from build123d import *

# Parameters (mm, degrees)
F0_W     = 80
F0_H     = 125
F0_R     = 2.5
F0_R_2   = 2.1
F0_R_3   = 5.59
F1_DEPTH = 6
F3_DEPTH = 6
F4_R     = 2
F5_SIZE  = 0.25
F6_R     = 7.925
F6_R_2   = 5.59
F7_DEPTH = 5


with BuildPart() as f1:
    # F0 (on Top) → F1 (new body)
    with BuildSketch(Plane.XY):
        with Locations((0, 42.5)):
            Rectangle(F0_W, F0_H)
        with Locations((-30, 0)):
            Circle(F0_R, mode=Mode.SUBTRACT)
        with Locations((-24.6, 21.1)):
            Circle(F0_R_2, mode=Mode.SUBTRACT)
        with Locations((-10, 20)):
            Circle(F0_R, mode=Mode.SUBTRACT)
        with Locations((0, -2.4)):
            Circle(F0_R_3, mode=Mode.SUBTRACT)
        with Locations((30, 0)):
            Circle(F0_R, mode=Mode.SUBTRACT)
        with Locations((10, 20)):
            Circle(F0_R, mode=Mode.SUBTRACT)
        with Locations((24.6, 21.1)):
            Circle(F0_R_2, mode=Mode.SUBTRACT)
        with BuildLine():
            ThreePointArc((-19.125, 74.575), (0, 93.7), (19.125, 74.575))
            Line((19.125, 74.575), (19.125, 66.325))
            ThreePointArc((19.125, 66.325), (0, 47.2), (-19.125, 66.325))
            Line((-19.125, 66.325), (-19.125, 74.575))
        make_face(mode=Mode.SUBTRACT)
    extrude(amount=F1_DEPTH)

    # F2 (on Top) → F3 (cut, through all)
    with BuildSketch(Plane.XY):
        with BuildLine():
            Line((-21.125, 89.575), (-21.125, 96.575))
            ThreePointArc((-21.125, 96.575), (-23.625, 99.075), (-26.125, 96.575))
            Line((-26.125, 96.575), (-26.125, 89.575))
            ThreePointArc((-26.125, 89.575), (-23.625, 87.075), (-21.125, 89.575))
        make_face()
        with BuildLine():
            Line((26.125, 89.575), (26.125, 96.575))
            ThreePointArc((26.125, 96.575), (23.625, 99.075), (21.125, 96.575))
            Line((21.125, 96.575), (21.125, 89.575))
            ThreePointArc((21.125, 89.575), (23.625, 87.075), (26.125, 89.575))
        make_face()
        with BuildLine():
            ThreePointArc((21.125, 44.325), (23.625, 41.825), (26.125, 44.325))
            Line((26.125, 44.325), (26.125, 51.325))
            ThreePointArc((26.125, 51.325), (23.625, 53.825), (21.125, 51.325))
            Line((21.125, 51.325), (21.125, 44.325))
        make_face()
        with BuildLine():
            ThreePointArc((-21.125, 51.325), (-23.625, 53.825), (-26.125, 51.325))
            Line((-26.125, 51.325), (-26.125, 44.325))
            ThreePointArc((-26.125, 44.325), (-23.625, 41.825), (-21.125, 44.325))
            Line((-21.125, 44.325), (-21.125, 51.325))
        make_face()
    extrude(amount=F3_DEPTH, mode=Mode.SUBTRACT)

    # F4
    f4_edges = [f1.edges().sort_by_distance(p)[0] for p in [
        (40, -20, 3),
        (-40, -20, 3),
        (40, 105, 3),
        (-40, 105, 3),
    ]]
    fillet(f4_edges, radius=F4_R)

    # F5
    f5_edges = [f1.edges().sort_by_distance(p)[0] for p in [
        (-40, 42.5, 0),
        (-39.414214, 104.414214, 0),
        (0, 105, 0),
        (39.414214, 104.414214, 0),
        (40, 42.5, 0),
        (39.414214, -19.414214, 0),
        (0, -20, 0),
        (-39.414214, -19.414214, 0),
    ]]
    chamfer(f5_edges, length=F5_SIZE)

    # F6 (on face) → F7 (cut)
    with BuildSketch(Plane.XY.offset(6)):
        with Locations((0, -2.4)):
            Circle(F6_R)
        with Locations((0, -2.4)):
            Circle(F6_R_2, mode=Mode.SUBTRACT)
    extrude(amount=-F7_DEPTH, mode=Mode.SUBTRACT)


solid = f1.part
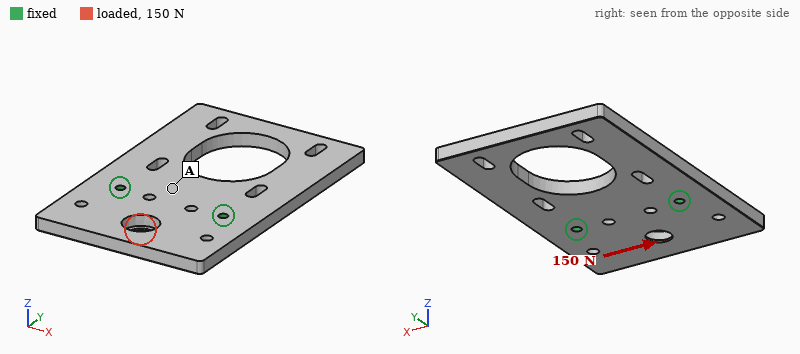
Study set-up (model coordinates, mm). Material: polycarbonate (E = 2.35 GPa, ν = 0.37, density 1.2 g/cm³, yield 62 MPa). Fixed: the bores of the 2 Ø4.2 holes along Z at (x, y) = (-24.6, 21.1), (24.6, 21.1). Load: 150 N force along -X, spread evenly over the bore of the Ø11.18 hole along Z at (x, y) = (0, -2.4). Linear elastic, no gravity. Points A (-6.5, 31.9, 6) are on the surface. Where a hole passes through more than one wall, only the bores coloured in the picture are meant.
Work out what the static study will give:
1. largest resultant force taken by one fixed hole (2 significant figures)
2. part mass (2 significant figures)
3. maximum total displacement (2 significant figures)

100 N
58 g
45 µm
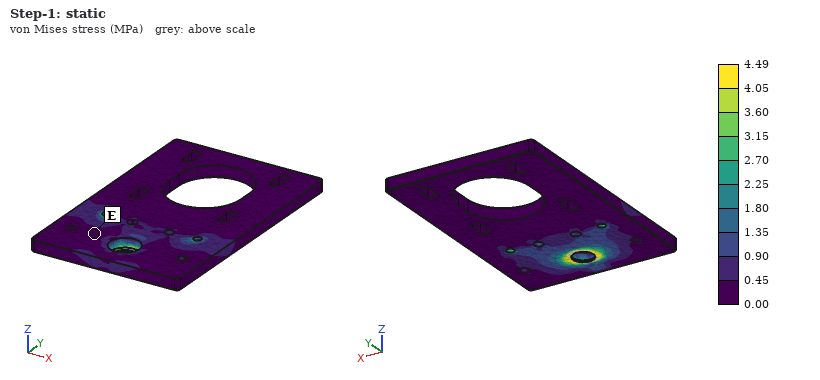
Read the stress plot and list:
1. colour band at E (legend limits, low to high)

0.00 to 0.45 MPa
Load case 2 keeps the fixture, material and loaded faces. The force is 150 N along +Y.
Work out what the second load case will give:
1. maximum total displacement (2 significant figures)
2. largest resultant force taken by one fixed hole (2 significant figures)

0.11 mm
78 N
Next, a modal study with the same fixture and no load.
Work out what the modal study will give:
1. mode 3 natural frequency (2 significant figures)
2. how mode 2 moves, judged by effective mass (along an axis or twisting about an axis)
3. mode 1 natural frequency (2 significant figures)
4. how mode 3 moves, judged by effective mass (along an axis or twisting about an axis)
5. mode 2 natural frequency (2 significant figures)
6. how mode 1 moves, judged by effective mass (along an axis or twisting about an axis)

680 Hz
twisting about Y
180 Hz
along Z
390 Hz
along Z
